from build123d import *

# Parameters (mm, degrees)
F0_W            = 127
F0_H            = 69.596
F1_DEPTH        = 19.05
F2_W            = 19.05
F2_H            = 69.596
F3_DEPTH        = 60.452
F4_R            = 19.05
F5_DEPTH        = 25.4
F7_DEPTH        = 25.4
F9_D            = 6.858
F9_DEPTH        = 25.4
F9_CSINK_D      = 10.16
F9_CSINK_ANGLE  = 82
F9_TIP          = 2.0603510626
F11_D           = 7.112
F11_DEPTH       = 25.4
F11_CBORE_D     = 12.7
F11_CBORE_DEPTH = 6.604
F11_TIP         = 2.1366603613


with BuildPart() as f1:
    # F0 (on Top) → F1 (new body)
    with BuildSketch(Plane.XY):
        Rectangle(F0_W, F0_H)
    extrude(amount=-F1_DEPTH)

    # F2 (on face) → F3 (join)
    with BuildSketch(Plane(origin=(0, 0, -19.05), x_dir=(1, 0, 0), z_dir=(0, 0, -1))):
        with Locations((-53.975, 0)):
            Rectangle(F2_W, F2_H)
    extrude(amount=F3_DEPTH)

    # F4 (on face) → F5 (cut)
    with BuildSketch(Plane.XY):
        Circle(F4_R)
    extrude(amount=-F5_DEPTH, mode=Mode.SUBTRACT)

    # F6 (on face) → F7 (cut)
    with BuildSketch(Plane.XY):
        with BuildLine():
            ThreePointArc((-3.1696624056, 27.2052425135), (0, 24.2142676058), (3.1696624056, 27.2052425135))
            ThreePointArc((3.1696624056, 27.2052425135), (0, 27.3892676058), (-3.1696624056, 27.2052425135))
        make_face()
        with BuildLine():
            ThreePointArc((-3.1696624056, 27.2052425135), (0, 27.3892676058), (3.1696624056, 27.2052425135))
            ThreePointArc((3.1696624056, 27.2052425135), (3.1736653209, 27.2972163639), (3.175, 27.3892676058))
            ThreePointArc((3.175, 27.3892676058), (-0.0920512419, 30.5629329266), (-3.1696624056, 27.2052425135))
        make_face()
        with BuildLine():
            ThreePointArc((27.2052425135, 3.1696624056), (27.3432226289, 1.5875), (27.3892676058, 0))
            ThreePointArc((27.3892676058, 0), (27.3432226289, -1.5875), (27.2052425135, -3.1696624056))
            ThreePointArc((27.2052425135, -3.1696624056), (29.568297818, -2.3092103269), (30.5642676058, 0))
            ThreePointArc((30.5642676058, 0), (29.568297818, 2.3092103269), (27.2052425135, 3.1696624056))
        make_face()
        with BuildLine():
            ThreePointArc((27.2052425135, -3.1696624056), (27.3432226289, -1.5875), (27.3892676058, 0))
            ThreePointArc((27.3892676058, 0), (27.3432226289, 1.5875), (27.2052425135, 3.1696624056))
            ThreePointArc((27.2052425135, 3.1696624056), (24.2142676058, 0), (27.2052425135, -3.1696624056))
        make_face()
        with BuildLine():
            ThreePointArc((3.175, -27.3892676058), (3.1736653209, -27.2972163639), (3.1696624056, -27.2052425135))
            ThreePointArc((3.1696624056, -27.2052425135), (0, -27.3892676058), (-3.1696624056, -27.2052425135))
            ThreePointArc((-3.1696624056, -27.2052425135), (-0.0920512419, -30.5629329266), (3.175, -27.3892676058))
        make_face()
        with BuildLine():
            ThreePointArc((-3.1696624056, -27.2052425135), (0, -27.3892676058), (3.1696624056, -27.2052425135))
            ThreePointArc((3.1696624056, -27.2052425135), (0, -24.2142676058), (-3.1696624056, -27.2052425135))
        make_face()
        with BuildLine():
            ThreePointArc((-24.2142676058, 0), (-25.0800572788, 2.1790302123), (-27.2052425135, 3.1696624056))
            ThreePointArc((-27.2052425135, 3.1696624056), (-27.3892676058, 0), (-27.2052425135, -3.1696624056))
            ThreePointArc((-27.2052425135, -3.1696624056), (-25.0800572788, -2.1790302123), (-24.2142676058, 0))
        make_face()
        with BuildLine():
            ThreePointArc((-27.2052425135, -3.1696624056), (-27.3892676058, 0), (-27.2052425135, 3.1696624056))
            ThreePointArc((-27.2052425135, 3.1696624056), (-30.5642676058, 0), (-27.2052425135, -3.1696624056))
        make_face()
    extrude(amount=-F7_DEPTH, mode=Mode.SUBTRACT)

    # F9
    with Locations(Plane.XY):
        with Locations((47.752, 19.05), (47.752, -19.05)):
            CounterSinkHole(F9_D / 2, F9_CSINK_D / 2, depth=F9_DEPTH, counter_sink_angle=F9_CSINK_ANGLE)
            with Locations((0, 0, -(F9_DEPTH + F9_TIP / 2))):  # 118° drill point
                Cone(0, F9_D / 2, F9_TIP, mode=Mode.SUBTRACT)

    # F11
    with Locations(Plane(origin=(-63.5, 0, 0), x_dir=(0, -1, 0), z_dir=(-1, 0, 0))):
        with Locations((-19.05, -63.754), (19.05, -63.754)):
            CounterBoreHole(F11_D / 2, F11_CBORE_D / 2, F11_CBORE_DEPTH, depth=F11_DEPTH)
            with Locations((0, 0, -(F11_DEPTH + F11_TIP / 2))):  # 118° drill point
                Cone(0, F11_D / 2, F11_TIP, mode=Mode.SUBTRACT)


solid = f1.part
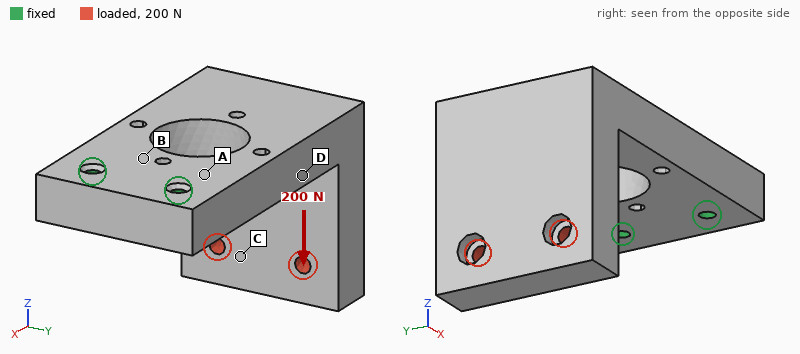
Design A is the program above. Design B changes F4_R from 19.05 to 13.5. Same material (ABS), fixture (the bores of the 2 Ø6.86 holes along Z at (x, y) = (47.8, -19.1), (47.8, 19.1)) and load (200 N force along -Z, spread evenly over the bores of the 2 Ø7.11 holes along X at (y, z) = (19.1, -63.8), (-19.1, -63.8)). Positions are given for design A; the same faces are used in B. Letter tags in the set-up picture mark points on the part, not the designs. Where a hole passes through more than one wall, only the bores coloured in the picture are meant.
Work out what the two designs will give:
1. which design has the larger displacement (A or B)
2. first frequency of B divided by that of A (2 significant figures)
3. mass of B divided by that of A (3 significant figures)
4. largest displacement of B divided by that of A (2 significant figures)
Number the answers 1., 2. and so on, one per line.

1. A
2. 1.1
3. 1.05
4. 0.81
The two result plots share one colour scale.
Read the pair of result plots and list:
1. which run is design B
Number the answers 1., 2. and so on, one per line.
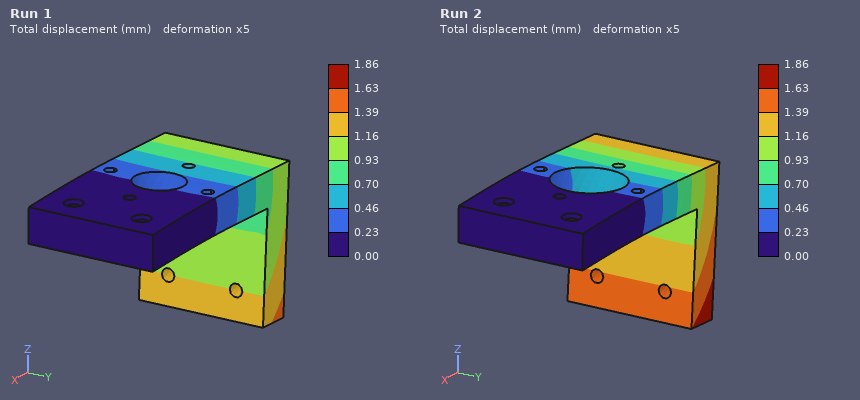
1. Run 1
